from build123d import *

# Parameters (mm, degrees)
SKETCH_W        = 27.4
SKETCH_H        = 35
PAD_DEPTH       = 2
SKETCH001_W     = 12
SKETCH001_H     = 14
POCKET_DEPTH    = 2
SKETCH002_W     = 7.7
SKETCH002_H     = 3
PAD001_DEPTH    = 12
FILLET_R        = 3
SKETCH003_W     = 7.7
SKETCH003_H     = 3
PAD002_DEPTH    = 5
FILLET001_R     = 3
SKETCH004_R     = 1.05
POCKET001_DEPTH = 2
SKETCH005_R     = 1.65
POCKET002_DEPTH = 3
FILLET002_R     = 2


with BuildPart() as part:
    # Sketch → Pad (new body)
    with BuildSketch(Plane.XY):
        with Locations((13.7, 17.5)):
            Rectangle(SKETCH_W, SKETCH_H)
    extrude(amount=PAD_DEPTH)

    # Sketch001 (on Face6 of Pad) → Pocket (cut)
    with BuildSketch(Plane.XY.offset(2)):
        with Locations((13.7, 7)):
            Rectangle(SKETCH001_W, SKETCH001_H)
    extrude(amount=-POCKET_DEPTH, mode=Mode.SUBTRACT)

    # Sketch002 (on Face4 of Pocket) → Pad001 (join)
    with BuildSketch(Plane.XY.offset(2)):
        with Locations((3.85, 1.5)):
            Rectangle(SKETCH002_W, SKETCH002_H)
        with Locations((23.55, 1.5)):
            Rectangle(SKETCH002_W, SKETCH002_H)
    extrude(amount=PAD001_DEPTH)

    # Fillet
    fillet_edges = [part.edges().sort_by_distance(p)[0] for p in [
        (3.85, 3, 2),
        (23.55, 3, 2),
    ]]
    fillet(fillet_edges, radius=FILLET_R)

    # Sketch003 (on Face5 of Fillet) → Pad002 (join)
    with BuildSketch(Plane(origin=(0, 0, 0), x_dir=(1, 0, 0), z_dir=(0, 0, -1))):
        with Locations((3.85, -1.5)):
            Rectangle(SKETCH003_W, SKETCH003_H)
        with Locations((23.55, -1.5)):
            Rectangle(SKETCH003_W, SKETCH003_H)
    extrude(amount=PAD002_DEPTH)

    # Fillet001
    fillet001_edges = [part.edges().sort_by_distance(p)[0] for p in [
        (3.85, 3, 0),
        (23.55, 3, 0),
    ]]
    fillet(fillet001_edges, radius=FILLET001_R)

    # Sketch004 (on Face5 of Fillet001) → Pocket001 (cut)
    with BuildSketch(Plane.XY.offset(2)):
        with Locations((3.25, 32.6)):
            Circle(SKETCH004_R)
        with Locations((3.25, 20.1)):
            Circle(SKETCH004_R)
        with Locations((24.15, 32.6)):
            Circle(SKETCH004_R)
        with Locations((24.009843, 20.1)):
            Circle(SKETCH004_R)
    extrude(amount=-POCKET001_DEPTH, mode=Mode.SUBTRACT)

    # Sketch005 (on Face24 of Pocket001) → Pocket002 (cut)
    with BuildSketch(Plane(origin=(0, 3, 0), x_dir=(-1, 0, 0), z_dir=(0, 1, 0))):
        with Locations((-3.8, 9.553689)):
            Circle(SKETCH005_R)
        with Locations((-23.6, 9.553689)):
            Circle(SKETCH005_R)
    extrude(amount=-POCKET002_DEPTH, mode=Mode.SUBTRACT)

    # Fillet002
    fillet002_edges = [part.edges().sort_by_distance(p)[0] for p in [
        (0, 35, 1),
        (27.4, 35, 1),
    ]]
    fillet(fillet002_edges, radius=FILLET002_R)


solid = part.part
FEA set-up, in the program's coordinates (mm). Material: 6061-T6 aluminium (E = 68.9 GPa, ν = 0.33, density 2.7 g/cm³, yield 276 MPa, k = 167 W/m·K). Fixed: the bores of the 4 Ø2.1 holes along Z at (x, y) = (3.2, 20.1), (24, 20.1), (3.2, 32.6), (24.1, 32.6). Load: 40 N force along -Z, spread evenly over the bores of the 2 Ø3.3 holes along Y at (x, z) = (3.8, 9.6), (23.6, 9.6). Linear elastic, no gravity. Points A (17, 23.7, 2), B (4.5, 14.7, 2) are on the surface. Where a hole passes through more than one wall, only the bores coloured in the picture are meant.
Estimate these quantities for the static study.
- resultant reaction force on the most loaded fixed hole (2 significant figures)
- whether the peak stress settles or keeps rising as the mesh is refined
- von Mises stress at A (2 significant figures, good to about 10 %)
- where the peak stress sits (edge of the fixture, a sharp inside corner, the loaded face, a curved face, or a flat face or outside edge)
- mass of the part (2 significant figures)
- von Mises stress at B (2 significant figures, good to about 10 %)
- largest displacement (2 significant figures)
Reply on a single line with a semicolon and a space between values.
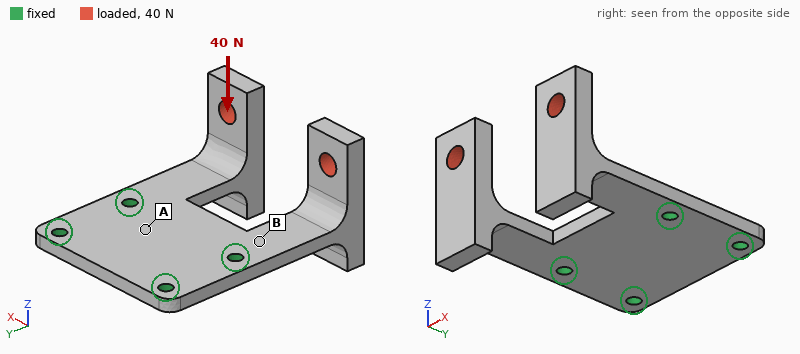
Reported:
28 N; keeps rising; 7.7 MPa; edge of the fixture; 6.3 g; 44 MPa; 0.15 mm
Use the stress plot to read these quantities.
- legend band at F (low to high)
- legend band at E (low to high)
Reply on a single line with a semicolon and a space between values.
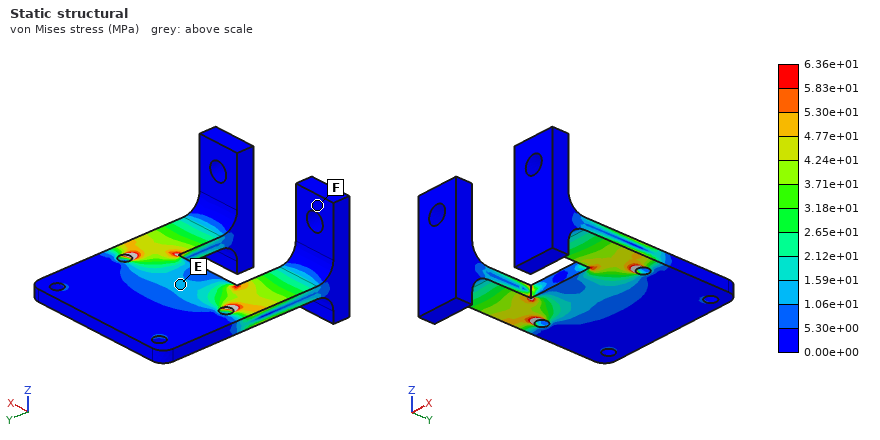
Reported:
0.00e+00 to 5.30e+00 MPa; 1.06e+01 to 1.59e+01 MPa
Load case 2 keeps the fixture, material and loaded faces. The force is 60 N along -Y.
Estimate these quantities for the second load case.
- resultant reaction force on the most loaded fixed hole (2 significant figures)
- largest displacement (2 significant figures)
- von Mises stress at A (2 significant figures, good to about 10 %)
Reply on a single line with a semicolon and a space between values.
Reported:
27 N; 0.18 mm; 5.8 MPa
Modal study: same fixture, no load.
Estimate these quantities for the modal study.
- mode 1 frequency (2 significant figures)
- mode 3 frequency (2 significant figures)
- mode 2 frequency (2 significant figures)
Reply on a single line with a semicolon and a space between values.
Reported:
1800 Hz; 4000 Hz; 1800 Hz
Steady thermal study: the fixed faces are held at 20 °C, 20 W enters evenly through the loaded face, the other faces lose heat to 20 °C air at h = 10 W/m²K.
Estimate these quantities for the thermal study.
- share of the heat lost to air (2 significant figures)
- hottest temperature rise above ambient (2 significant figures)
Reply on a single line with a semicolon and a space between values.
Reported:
3.9 %; 83 K
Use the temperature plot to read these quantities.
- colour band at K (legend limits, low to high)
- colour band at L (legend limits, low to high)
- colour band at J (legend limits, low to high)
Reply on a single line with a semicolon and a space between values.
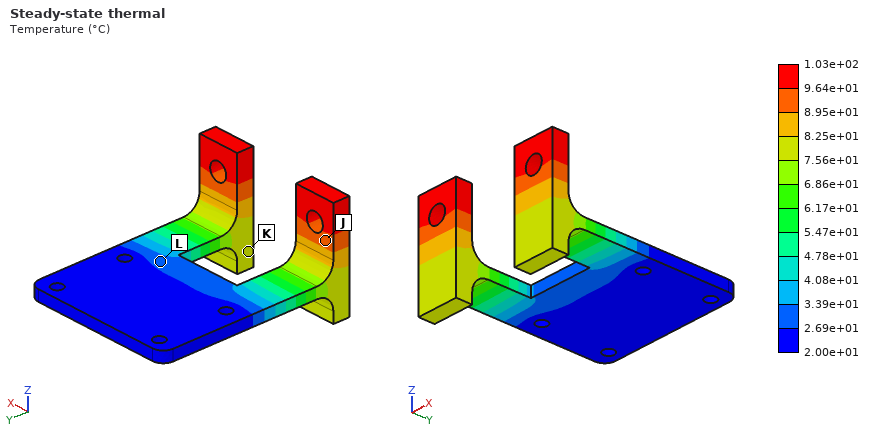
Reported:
7.56e+01 to 8.25e+01 °C; 2.69e+01 to 3.39e+01 °C; 8.95e+01 to 9.64e+01 °C
